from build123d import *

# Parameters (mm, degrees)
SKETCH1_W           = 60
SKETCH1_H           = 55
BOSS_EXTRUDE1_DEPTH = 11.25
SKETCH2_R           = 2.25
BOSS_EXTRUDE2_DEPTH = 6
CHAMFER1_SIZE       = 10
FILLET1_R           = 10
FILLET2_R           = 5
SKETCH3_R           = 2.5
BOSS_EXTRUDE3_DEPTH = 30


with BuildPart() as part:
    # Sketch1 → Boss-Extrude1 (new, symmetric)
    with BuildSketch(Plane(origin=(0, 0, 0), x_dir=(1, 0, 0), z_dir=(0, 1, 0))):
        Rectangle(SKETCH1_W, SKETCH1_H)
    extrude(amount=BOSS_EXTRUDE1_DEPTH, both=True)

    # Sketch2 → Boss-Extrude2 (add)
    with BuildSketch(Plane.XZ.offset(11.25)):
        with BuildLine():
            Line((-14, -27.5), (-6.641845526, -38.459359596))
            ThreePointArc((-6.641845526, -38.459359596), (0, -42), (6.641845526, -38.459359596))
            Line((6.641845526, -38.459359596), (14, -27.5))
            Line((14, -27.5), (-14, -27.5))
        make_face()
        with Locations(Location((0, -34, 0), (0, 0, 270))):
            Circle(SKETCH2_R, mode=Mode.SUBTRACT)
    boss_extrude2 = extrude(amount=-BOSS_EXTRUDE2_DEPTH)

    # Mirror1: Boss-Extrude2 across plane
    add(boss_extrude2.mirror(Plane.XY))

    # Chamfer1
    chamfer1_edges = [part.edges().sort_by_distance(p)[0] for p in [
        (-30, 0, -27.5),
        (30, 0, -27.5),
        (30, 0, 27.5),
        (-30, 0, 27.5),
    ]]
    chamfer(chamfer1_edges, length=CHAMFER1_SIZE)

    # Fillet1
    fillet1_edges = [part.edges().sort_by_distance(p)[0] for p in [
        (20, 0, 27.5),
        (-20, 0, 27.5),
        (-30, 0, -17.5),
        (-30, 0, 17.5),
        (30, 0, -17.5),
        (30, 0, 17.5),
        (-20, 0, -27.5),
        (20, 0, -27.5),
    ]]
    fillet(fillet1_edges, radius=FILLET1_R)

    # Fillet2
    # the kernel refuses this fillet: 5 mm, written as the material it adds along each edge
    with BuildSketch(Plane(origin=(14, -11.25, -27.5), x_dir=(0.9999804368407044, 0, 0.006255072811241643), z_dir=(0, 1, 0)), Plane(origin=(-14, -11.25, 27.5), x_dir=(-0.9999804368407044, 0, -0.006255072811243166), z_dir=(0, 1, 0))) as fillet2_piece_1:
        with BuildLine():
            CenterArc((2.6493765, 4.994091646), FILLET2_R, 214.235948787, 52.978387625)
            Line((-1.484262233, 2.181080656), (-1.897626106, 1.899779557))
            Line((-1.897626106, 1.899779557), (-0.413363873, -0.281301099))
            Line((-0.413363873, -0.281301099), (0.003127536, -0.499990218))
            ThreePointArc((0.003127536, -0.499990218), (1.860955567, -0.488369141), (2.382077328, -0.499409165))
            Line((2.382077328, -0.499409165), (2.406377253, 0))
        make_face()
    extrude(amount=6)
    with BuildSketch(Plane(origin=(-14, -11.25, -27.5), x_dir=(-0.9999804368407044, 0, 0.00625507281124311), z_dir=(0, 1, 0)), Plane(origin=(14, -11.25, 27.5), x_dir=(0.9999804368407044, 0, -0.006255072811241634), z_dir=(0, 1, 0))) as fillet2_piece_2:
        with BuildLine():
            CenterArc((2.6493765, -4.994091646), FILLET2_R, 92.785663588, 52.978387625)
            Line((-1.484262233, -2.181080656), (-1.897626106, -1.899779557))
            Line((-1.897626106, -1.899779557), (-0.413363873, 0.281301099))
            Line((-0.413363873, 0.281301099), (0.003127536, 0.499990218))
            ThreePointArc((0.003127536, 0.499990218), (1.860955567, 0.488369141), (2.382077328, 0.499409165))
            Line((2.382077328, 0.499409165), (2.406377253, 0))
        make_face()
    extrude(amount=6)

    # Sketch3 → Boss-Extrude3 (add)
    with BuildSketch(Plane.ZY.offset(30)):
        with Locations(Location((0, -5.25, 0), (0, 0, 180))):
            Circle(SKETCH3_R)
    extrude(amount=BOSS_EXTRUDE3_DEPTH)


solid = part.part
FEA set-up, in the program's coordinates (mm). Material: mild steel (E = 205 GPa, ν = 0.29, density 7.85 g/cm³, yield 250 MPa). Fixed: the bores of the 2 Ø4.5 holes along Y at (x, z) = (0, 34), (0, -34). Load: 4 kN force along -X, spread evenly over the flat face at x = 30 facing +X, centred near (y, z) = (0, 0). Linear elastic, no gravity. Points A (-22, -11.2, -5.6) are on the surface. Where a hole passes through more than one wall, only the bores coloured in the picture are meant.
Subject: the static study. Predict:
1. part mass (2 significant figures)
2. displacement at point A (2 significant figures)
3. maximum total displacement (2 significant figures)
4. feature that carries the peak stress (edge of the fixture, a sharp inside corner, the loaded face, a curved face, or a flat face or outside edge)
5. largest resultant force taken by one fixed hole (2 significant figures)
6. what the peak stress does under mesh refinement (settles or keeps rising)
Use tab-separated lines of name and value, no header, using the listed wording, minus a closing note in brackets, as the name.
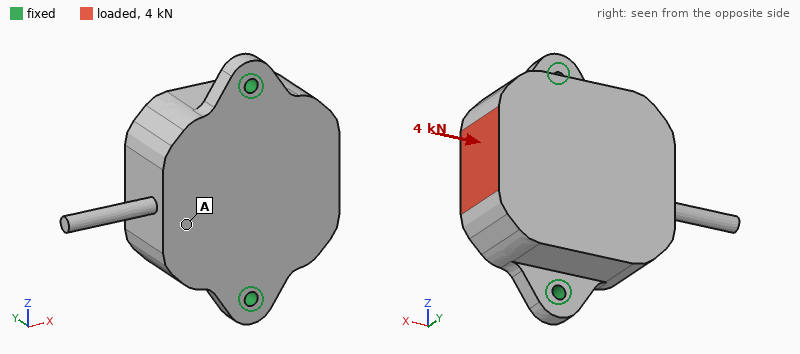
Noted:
part mass	570 g
displacement at point A	25 µm
maximum total displacement	69 µm
feature that carries the peak stress	edge of the fixture
largest resultant force taken by one fixed hole	2.0 kN
what the peak stress does under mesh refinement	keeps rising
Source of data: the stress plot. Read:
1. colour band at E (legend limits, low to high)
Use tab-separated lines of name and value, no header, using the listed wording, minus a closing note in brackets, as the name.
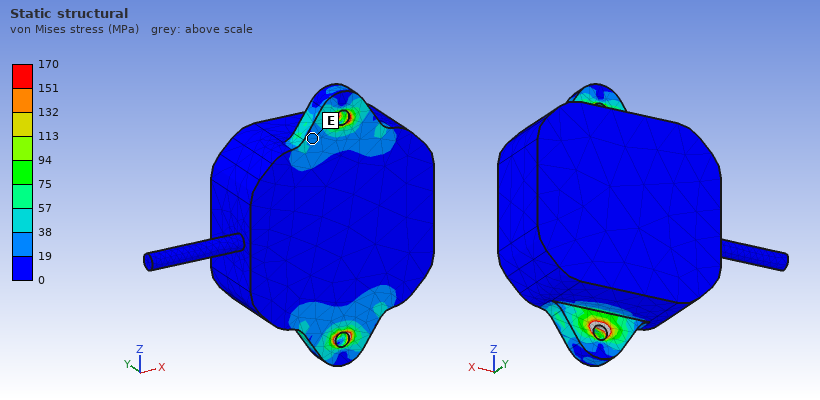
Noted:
colour band at E	19 to 38 MPa
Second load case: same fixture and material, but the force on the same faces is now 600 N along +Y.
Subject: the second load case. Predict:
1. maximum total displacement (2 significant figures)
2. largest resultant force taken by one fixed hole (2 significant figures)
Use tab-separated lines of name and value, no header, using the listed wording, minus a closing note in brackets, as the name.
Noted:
maximum total displacement	35 µm
largest resultant force taken by one fixed hole	360 N
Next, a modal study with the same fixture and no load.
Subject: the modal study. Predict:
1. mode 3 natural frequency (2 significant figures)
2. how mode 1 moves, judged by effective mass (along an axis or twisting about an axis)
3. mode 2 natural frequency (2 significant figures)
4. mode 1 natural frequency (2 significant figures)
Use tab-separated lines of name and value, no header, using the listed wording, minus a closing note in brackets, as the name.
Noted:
mode 3 natural frequency	3700 Hz
how mode 1 moves, judged by effective mass	along X
mode 2 natural frequency	3600 Hz
mode 1 natural frequency	1800 Hz
